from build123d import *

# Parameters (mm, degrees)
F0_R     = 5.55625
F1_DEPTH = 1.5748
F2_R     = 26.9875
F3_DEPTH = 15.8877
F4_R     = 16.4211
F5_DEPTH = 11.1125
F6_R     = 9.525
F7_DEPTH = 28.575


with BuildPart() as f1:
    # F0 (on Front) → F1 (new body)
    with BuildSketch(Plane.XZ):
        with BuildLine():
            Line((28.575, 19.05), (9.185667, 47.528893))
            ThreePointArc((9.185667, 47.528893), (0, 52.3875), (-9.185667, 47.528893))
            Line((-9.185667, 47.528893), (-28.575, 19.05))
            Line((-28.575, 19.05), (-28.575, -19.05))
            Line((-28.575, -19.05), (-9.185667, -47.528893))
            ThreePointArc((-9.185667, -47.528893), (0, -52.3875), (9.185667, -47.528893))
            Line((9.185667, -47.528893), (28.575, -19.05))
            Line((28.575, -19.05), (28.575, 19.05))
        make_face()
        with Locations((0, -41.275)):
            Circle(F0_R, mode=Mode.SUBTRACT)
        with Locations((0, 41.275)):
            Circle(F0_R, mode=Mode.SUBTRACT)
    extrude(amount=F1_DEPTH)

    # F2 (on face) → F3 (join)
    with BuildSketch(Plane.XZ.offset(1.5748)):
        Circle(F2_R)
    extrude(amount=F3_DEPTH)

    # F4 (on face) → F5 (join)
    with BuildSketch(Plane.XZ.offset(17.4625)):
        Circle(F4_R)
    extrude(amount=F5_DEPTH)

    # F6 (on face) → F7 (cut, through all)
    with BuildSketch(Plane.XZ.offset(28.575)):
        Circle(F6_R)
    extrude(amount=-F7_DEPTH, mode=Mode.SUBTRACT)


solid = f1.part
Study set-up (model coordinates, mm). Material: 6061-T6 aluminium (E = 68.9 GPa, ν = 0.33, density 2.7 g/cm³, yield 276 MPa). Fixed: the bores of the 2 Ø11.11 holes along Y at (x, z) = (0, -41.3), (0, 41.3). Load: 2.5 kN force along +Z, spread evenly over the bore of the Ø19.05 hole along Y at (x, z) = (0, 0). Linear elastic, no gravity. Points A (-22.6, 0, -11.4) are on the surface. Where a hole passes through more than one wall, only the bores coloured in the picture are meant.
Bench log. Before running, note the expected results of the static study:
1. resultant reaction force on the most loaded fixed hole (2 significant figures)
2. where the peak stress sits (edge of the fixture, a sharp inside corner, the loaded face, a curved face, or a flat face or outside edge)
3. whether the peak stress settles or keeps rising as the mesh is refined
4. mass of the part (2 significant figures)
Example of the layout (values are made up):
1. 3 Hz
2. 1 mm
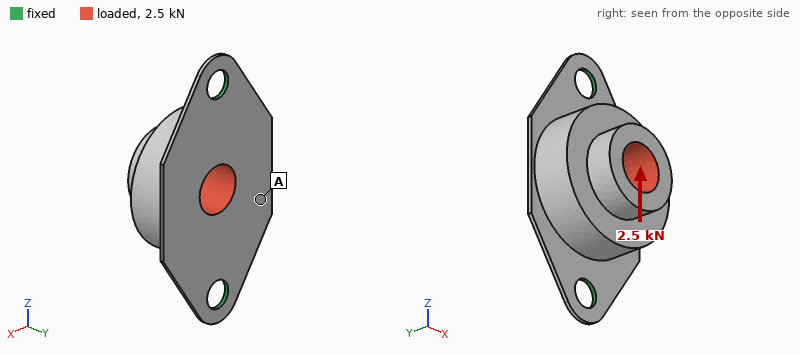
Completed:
1. 1.4 kN
2. edge of the fixture
3. keeps rising
4. 120 g
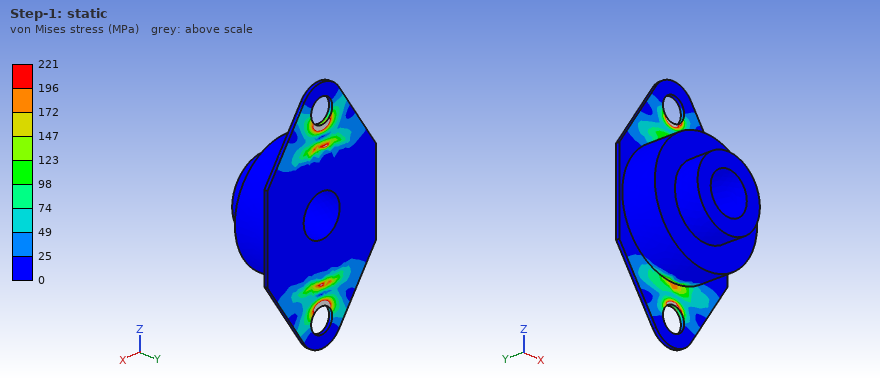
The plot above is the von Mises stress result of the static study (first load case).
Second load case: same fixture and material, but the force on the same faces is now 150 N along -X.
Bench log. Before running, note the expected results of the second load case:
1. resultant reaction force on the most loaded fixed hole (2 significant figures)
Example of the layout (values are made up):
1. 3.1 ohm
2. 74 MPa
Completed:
1. 75 N
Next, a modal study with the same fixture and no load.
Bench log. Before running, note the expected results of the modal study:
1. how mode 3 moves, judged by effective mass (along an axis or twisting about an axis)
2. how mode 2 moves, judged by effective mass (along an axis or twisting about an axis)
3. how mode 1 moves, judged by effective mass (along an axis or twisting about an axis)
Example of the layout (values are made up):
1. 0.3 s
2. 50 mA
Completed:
1. along Z
2. along Y
3. along X
